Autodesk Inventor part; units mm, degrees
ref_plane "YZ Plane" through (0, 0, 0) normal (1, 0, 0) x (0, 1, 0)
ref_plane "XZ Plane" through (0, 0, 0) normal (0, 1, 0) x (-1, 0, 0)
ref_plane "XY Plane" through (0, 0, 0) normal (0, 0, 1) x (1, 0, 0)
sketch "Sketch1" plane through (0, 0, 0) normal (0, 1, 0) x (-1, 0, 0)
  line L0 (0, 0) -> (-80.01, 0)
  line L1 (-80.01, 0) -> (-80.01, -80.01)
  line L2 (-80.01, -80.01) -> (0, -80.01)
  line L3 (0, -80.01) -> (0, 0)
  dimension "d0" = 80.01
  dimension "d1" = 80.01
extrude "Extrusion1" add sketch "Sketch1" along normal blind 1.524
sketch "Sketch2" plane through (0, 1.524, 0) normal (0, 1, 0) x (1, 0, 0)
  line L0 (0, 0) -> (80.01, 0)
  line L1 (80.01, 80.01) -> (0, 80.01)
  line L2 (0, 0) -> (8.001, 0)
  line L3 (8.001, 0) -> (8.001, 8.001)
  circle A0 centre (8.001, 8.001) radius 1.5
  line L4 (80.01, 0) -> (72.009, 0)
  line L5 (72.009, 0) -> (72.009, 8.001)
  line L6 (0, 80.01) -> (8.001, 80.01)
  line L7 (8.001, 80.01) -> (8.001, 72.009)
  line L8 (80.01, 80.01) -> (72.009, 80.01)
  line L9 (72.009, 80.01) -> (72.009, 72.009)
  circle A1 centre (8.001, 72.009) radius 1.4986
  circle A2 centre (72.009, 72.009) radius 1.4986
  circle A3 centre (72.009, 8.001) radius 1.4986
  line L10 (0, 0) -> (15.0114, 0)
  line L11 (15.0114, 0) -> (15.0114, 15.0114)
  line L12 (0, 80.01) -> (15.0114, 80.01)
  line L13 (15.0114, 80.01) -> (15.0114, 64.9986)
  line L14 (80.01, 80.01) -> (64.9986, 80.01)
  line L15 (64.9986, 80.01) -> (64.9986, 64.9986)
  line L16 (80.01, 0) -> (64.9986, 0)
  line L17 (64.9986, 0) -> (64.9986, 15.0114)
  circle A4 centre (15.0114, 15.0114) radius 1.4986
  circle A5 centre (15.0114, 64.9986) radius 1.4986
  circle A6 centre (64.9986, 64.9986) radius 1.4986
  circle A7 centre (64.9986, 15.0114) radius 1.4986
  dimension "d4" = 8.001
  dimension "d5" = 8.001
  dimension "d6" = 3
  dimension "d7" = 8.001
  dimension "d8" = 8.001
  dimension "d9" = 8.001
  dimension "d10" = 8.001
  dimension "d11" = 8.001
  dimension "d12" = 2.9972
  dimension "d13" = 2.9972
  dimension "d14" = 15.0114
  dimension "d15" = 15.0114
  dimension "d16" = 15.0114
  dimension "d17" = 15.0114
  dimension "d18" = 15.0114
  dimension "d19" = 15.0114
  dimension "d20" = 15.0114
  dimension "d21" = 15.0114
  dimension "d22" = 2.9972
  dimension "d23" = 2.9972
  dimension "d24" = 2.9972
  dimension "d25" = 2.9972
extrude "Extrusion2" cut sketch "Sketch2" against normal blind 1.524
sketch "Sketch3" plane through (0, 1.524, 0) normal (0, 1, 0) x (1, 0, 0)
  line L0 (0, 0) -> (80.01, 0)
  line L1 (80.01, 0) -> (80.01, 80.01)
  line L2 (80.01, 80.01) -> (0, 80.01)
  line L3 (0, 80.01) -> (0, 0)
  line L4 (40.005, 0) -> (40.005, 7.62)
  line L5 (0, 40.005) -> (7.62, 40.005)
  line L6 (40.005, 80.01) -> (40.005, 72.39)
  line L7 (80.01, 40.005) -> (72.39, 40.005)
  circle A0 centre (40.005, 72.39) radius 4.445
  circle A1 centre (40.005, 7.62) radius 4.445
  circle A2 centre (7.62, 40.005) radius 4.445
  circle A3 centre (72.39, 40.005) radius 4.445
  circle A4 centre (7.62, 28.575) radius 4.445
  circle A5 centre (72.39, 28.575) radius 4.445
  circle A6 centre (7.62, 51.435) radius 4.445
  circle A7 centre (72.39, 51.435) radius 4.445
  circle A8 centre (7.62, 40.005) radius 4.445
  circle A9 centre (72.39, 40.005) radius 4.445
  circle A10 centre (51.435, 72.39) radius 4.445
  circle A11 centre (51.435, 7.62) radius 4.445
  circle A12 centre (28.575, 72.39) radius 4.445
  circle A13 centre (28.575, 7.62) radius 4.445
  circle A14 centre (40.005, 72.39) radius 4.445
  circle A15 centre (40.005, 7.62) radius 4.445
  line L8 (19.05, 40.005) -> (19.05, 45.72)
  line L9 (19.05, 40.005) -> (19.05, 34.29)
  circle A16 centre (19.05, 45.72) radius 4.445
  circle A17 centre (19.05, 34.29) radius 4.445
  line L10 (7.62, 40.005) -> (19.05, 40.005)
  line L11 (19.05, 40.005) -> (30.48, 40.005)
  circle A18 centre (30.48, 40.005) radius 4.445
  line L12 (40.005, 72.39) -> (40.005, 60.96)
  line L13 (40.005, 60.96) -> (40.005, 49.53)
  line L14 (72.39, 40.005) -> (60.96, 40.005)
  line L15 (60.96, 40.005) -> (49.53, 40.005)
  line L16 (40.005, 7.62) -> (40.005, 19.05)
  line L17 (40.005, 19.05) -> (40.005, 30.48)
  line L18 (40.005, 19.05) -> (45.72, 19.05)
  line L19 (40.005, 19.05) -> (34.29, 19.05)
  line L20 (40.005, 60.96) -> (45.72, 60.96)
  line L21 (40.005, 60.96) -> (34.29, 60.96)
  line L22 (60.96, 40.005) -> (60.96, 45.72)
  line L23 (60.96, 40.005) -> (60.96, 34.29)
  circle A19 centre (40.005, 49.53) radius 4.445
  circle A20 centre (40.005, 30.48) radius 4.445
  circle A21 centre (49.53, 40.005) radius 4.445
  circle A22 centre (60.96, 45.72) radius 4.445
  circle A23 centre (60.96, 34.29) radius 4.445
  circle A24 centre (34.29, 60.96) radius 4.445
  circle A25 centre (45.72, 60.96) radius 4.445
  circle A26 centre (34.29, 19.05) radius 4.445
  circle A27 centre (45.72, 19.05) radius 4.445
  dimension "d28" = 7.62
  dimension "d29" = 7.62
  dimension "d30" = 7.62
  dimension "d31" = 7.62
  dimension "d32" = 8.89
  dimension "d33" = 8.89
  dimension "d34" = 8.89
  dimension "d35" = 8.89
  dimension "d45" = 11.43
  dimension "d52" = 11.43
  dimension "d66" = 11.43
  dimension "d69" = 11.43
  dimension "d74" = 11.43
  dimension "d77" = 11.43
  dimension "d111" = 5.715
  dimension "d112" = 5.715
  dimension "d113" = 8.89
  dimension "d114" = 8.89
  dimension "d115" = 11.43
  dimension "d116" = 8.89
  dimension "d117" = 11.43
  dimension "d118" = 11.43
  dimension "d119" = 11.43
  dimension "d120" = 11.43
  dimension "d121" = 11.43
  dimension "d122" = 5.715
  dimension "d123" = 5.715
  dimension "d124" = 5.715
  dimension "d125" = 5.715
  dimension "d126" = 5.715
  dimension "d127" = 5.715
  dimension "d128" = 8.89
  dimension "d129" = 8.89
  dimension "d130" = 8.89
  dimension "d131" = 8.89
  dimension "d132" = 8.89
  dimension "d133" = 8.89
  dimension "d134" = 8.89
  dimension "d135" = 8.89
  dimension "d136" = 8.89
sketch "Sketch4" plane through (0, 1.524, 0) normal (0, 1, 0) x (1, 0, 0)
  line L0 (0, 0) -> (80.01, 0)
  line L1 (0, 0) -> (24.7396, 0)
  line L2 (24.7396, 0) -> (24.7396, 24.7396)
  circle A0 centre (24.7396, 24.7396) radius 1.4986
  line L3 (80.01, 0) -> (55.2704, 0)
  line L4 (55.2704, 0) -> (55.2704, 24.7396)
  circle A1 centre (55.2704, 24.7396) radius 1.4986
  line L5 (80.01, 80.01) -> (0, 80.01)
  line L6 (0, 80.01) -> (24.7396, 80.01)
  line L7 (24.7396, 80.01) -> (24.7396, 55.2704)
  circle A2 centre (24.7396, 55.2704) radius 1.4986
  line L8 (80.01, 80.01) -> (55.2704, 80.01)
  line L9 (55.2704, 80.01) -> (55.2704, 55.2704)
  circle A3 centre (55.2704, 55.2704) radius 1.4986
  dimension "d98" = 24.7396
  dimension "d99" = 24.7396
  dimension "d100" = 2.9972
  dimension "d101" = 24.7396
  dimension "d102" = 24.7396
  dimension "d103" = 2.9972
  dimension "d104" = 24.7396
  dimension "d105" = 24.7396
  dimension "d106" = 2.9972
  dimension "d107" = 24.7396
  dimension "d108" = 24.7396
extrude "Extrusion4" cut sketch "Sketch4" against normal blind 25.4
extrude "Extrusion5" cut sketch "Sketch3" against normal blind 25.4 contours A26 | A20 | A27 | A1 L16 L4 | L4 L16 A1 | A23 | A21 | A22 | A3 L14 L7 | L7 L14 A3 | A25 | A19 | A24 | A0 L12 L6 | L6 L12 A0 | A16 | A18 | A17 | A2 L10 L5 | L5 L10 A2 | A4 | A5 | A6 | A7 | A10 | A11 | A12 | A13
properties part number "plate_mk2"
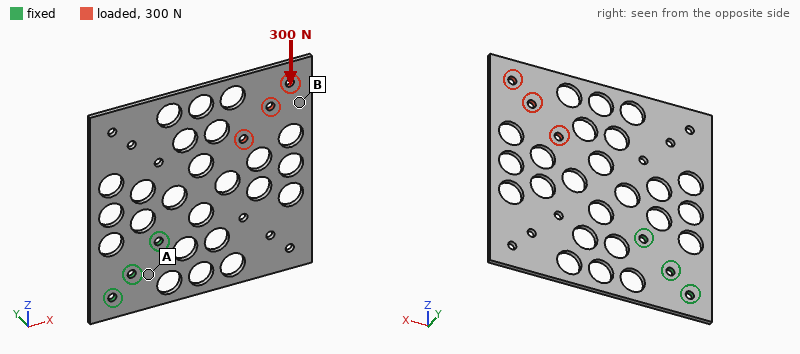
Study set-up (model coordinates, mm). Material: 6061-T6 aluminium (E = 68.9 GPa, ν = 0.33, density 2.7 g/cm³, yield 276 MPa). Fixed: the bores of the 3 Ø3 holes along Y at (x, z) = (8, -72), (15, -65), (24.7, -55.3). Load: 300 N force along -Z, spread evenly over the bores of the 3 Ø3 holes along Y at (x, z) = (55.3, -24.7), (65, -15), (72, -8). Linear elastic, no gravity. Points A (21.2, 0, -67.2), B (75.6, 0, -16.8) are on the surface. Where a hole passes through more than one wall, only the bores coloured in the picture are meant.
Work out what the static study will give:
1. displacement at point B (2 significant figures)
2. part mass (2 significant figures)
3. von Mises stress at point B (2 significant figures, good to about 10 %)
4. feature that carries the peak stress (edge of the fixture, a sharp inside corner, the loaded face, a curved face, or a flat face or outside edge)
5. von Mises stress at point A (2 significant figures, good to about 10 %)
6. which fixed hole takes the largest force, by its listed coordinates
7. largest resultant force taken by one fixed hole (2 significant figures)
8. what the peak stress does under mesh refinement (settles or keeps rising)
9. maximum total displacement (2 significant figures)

0.095 mm
20 g
4.9 MPa
edge of the fixture
18 MPa
(24.7, -55.3)
700 N
keeps rising
0.11 mm
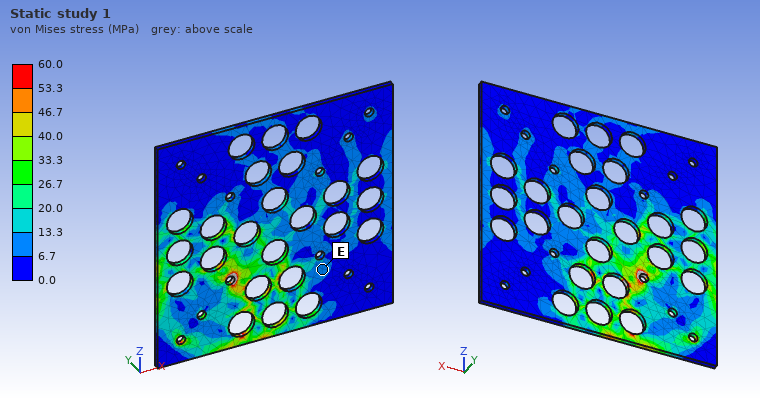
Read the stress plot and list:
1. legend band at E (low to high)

6.7 to 13.3 MPa
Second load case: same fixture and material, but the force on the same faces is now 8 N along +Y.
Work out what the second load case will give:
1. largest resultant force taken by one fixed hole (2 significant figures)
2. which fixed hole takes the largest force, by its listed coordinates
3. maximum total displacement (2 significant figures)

22 N
(24.7, -55.3)
1.1 mm
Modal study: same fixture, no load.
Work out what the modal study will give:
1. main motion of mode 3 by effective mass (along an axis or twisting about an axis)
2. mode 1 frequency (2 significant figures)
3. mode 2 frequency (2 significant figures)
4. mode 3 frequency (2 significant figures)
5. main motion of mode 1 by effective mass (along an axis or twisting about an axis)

along Y
230 Hz
320 Hz
590 Hz
along Y
